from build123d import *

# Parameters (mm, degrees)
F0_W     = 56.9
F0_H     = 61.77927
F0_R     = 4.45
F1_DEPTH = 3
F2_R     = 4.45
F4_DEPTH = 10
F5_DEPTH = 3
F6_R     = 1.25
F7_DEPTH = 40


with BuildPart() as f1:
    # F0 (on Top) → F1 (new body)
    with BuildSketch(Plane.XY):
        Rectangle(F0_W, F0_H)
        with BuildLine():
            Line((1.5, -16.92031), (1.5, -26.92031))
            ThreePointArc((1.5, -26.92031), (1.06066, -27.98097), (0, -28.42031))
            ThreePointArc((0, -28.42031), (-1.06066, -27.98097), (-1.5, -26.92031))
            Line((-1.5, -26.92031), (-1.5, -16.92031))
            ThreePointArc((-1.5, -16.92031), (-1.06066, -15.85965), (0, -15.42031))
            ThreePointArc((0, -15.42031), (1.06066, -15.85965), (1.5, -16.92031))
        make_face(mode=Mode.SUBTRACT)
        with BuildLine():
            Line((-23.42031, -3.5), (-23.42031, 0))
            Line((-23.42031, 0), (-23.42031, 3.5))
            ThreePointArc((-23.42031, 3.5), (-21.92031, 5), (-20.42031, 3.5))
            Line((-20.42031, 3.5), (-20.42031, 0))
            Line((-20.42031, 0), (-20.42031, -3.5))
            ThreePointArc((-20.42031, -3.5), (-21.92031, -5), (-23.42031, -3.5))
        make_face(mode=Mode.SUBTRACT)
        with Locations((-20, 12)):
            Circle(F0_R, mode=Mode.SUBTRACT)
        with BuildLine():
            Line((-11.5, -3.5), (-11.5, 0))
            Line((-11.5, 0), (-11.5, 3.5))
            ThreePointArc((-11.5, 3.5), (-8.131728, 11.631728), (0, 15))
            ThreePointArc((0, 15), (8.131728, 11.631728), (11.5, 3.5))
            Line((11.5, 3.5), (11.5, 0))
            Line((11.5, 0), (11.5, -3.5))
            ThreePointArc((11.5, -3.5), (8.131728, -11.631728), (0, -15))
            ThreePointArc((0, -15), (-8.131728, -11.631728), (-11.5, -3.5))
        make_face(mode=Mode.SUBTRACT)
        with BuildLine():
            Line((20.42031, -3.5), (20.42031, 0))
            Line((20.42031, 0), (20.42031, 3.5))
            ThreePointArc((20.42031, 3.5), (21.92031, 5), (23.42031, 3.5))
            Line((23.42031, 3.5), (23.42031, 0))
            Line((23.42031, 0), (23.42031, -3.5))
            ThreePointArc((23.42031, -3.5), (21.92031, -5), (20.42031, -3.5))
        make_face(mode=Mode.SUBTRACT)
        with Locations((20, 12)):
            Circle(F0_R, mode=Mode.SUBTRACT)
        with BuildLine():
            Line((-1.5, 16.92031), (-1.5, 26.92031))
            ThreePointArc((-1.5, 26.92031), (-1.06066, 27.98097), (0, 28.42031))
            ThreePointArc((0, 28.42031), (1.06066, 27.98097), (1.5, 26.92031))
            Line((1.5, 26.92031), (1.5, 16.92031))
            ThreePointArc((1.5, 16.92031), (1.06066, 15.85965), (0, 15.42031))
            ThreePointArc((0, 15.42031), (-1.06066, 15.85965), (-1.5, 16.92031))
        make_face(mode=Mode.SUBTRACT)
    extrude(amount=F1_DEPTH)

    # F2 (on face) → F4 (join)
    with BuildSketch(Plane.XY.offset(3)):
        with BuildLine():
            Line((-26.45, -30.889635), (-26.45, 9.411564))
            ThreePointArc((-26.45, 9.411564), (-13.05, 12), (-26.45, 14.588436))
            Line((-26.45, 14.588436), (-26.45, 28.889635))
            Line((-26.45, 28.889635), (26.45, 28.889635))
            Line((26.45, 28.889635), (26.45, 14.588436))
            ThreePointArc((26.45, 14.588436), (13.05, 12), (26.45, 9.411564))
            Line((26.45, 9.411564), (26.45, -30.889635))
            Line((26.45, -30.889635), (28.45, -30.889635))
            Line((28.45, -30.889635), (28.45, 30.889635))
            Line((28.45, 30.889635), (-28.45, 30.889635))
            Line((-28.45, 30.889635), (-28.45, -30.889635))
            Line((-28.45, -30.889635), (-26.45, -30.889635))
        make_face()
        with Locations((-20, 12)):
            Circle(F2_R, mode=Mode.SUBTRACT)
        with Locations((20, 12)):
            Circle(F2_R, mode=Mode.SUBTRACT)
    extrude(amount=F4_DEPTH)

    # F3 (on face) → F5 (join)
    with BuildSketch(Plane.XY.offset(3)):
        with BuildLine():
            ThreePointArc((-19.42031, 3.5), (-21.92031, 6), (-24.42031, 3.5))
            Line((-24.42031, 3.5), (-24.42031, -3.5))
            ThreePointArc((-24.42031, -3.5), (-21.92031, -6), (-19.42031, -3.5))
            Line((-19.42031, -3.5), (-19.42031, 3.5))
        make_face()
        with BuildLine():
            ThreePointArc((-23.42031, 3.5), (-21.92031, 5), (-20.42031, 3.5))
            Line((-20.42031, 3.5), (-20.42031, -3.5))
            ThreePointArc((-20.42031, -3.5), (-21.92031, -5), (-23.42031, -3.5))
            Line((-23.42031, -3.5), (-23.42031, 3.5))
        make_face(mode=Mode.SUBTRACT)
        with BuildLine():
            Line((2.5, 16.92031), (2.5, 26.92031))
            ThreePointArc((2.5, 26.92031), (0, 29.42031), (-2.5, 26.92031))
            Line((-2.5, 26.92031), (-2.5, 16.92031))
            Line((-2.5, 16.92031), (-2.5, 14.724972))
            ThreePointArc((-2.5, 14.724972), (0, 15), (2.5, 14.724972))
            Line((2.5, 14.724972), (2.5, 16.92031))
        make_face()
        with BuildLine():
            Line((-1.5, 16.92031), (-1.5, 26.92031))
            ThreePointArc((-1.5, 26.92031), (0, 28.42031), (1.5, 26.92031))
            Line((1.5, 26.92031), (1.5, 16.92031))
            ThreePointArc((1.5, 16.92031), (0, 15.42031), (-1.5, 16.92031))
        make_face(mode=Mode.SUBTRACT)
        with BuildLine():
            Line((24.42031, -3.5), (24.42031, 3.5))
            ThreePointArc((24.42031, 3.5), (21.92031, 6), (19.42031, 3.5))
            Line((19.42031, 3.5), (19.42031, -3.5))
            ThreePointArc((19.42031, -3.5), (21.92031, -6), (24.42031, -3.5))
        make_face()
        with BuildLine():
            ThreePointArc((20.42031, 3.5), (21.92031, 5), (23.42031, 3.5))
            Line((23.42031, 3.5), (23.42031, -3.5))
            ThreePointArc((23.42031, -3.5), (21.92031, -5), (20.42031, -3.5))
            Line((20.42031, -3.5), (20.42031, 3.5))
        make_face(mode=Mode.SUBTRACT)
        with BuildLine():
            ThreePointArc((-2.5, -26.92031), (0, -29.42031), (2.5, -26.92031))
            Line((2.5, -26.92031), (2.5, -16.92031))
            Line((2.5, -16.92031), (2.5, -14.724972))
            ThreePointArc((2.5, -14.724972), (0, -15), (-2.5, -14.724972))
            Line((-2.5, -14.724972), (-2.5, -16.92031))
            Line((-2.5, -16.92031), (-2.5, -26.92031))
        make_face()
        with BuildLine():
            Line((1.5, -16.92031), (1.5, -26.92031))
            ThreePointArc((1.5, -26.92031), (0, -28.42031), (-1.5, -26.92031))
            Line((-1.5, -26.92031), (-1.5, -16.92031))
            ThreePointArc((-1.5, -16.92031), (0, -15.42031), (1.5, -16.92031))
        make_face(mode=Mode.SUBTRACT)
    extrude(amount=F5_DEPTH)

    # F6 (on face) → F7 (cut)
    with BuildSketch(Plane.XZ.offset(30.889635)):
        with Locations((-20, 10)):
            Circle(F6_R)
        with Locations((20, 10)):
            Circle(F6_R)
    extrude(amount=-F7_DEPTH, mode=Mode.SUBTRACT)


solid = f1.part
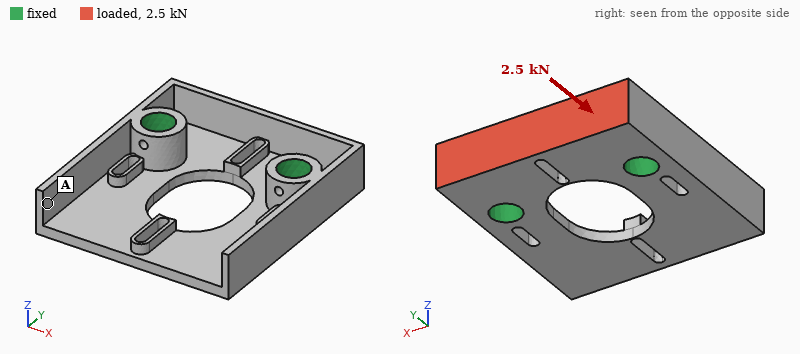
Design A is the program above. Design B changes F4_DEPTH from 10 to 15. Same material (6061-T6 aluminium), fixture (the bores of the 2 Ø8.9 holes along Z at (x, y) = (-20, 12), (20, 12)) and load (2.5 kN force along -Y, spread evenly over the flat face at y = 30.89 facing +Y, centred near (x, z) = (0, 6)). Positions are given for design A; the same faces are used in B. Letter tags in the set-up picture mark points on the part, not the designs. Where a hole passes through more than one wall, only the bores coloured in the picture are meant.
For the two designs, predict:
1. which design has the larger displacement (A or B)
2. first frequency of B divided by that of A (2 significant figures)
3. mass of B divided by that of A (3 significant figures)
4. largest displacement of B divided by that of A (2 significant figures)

B
1.0
1.19
1.9
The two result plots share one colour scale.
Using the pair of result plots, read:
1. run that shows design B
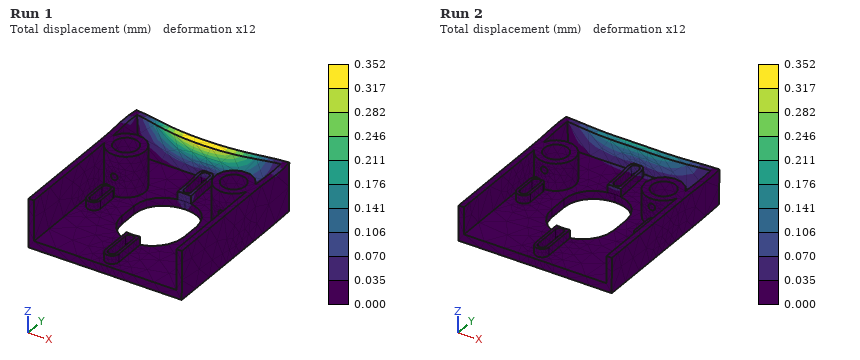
Run 1
